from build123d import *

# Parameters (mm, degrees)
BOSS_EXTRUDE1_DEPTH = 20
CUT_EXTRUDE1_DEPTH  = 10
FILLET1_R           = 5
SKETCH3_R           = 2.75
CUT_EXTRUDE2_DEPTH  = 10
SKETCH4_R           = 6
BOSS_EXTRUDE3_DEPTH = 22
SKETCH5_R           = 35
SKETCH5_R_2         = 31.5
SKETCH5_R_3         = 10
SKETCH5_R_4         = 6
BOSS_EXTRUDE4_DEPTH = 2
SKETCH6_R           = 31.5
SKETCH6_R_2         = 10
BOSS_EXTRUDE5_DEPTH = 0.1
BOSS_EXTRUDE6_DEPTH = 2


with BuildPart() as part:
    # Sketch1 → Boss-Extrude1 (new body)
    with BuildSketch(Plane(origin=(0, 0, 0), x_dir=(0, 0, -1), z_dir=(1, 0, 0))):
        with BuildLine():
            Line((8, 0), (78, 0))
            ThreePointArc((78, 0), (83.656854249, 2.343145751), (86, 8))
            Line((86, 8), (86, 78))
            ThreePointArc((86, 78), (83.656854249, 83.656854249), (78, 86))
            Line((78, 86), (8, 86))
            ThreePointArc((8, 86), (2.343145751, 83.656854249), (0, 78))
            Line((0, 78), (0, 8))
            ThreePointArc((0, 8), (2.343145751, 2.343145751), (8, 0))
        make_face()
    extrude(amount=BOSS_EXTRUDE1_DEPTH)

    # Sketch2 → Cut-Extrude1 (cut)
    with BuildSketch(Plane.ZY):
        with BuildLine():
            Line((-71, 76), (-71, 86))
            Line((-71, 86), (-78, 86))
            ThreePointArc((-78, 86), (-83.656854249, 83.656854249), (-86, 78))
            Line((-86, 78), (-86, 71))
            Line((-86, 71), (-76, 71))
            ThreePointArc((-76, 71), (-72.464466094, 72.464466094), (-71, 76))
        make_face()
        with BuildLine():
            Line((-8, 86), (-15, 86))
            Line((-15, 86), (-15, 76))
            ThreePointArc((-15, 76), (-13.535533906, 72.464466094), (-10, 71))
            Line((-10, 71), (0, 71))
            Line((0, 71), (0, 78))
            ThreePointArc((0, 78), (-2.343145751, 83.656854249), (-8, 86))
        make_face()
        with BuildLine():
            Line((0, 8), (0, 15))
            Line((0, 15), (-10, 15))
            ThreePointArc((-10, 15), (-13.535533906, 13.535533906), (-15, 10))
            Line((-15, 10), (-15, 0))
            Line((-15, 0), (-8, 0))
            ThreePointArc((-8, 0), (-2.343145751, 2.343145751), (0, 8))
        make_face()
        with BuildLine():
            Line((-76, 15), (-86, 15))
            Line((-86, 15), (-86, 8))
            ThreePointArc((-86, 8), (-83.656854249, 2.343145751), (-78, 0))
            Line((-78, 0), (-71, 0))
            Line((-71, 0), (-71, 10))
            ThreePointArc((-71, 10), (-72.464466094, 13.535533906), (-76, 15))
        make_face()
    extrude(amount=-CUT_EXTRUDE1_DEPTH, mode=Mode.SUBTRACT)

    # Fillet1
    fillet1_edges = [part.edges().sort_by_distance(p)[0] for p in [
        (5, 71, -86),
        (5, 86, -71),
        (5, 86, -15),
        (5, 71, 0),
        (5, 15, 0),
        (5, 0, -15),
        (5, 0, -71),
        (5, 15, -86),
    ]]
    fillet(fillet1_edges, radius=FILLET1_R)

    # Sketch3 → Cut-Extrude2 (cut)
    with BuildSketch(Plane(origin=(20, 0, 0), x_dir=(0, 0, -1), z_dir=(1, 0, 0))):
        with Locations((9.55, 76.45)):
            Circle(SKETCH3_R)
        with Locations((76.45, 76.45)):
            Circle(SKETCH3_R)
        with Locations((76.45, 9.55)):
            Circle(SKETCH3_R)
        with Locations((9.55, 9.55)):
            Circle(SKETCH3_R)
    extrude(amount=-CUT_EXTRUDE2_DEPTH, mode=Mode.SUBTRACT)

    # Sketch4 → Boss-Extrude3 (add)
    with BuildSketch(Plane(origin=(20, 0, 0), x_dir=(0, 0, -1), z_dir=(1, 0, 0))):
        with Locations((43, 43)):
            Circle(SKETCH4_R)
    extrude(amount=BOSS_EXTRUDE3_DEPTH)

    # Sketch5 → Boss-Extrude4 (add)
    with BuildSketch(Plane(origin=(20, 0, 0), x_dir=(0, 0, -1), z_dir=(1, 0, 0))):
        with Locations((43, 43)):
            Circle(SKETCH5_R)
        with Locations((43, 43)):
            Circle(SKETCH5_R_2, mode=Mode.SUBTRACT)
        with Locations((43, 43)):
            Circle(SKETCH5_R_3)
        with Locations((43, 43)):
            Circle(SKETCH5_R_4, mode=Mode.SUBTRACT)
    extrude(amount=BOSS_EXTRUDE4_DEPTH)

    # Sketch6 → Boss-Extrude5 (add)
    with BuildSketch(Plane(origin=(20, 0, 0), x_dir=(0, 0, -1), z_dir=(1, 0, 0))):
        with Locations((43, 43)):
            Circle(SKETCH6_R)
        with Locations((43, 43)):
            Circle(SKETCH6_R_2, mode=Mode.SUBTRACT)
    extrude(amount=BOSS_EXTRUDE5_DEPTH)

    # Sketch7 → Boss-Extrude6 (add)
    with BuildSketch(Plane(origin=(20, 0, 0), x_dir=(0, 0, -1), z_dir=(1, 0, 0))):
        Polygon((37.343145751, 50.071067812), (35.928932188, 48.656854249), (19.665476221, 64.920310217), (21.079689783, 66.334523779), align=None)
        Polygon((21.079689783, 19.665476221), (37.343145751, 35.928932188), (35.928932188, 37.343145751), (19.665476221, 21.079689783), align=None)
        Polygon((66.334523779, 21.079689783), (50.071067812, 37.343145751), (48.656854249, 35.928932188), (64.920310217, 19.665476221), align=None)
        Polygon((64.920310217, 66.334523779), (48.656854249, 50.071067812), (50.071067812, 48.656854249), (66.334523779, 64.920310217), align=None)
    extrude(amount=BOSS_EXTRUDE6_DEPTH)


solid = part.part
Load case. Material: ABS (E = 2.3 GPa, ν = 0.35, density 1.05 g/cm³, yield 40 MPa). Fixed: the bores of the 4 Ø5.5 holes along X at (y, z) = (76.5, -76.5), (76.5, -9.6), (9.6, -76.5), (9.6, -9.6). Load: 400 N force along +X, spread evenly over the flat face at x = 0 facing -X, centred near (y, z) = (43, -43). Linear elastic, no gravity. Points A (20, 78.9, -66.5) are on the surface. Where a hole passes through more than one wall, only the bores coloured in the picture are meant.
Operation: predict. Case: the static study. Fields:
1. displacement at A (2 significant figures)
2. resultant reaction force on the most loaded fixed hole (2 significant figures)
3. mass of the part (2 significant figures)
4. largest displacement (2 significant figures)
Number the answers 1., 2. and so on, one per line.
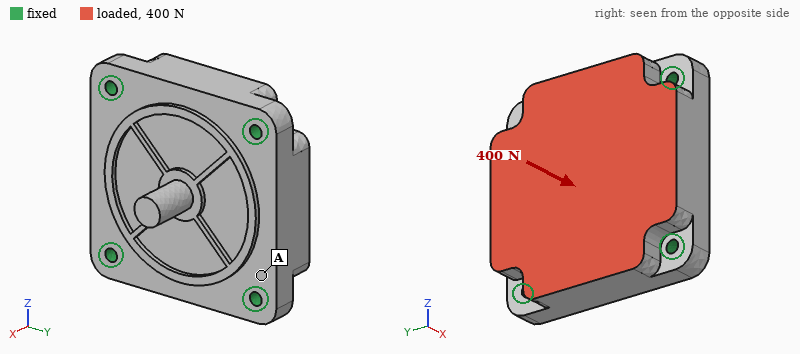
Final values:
1. 5.6 µm
2. 110 N
3. 150 g
4. 14 µm
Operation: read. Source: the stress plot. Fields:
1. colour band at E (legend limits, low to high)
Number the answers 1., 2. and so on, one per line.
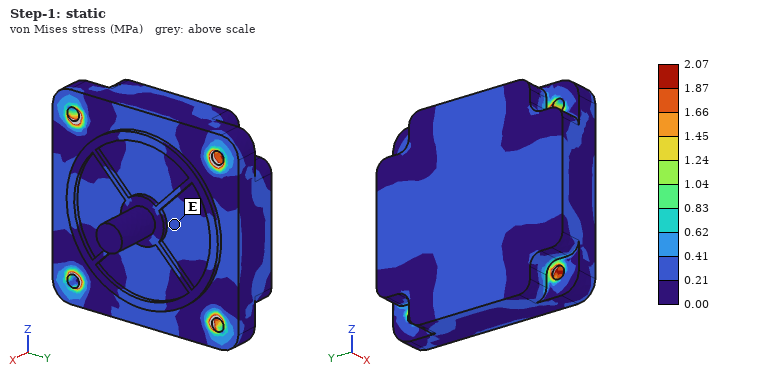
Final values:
1. 0.21 to 0.41 MPa
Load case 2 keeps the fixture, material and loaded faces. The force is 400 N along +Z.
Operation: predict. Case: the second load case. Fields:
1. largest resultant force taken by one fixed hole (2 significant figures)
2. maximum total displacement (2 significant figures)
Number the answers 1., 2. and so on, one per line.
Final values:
1. 110 N
2. 9.8 µm
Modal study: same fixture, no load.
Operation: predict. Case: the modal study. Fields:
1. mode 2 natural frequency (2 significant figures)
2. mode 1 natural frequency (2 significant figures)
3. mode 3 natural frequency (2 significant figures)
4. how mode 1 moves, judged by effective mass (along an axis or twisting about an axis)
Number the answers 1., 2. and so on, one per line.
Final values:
1. 3600 Hz
2. 2500 Hz
3. 3600 Hz
4. along X
